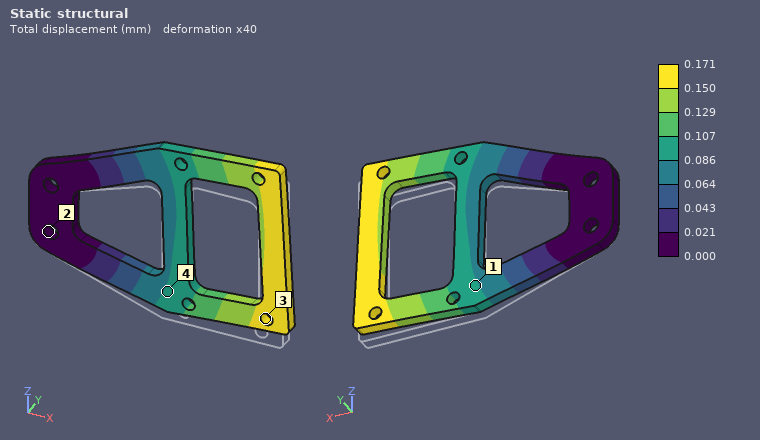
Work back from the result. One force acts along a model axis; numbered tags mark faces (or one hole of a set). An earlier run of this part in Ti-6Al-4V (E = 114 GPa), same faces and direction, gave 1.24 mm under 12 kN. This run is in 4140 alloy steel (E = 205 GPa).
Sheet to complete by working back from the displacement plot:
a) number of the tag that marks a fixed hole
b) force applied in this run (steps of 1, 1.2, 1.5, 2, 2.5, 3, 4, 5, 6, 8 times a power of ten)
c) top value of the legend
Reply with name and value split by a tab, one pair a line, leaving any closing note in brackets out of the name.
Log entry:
number of the tag that marks a fixed hole	2
force applied in this run	3 kN
top value of the legend	0.171 mm
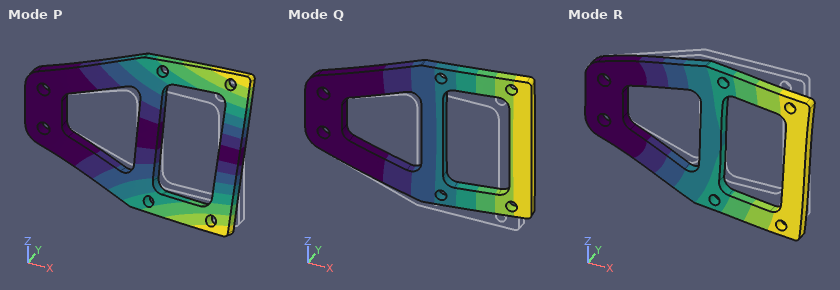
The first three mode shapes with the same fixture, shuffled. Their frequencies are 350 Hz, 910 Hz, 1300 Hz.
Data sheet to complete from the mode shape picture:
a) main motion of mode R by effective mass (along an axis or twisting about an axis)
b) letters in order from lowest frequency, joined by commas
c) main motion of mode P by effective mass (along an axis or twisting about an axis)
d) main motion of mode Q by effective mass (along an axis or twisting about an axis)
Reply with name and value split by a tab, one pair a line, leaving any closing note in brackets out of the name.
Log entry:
main motion of mode R by effective mass	along Z
letters in order from lowest frequency, joined by commas	Q, P, R
main motion of mode P by effective mass	twisting about X
main motion of mode Q by effective mass	along Y
